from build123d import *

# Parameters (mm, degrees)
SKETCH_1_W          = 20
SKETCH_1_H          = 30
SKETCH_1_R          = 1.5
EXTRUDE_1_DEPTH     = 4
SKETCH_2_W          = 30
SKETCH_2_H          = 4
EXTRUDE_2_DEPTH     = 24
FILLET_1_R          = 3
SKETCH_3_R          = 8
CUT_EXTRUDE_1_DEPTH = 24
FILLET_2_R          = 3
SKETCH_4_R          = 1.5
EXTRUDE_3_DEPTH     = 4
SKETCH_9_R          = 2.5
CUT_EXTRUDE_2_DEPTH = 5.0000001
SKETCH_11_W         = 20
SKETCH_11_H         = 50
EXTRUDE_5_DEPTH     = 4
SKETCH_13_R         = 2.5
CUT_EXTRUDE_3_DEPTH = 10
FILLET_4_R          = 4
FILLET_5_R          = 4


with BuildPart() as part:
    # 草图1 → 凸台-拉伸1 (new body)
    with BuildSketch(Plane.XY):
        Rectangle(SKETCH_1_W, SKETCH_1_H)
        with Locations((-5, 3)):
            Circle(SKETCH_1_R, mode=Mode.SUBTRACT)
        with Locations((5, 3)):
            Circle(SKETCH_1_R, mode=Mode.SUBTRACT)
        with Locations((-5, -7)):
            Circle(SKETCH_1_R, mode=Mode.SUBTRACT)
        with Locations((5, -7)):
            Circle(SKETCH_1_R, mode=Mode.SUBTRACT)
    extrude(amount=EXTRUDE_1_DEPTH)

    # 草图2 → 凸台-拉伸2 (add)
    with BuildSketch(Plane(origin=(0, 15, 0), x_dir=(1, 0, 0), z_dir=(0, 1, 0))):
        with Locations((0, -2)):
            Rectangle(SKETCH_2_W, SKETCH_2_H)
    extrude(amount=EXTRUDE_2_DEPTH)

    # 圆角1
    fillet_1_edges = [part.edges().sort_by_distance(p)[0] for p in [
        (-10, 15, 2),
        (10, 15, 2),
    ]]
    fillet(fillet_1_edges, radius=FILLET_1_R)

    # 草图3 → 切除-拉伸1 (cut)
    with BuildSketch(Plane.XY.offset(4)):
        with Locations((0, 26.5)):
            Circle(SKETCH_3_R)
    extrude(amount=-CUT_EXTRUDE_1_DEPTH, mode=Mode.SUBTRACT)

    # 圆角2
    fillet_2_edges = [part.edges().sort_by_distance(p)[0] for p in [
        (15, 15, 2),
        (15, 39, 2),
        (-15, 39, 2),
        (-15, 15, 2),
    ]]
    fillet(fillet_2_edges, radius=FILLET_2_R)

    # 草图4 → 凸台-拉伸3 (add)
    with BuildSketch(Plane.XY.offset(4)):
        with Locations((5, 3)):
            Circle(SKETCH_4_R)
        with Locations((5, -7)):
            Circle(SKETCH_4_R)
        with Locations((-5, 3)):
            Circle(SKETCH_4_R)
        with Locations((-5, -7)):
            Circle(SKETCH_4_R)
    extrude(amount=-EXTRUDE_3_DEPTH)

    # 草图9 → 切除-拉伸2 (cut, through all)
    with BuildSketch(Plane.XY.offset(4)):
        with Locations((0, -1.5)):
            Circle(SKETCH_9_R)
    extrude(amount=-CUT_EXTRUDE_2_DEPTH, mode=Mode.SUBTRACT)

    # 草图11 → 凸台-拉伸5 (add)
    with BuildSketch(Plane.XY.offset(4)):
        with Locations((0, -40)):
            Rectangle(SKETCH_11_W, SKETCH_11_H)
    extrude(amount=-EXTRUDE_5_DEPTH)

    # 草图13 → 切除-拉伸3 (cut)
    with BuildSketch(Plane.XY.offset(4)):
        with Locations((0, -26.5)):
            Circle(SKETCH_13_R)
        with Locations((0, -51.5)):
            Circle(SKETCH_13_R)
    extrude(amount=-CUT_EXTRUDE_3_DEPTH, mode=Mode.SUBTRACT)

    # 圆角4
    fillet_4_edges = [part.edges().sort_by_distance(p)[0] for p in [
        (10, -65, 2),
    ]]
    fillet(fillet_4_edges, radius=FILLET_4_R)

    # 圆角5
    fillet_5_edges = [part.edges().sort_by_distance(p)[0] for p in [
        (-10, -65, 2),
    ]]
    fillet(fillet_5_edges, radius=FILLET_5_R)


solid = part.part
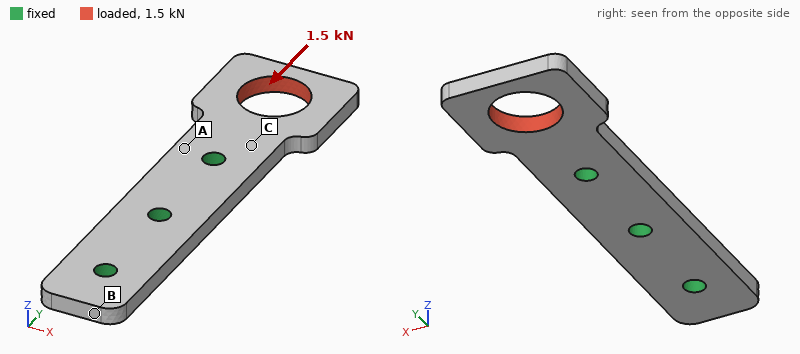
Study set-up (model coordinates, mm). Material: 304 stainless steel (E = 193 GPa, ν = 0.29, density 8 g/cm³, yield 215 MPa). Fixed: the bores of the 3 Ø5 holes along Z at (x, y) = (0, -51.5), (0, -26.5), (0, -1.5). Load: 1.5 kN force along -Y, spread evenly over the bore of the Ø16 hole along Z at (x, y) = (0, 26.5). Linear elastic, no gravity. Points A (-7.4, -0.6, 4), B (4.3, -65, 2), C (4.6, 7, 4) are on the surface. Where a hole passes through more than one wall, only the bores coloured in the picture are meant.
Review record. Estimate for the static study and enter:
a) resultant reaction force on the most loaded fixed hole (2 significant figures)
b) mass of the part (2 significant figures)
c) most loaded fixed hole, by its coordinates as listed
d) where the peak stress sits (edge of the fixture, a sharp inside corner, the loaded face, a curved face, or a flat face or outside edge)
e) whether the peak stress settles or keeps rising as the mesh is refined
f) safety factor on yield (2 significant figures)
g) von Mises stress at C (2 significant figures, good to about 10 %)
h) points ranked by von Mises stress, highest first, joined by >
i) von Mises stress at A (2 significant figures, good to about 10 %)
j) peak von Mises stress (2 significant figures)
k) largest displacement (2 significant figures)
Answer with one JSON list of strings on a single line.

["1.3 kN", "66 g", "(0, -1.5)", "a curved face", "settles", "3.6", "20 MPa", "C > A > B", "11 MPa", "61 MPa", "7.7 µm"]
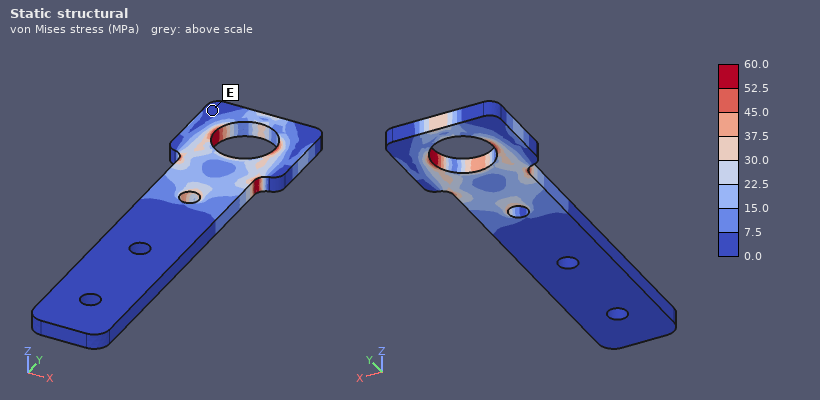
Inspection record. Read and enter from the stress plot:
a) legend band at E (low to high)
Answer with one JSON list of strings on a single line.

["0.0 to 7.5 MPa"]
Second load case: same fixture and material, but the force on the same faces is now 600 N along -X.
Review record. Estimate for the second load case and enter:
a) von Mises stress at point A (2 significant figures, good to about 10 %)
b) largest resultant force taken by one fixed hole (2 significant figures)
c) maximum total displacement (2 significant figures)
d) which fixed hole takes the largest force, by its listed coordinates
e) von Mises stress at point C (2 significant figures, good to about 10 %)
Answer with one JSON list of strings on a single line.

["38 MPa", "1.0 kN", "35 µm", "(0, -1.5)", "23 MPa"]
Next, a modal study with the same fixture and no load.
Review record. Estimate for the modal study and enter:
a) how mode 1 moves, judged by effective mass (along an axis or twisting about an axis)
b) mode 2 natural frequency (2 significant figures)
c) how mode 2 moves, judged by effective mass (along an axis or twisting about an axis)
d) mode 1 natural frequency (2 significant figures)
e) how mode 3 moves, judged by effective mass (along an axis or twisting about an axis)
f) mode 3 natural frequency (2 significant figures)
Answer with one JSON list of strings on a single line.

["along Z", "4200 Hz", "twisting about Y", "1900 Hz", "along X", "5600 Hz"]
